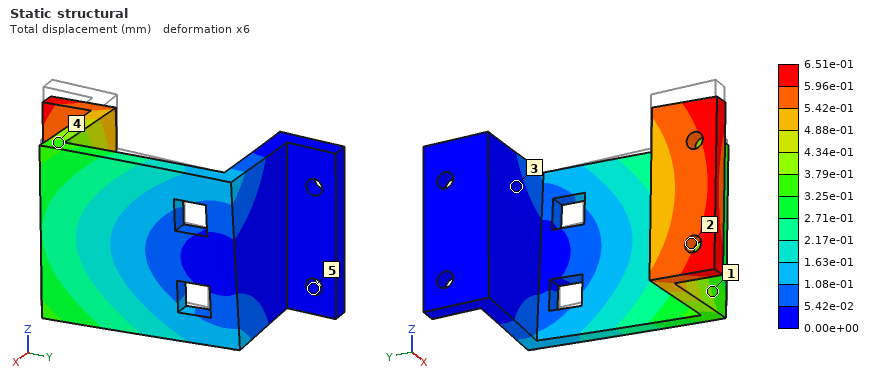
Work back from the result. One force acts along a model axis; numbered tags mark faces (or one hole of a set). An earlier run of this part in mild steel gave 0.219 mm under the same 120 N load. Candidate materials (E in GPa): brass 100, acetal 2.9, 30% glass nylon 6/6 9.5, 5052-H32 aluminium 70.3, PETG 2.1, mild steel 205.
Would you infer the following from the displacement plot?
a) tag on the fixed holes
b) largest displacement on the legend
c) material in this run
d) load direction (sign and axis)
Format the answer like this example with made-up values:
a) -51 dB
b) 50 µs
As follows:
a) 5
b) 6.51e-01 mm
c) 5052-H32 aluminium
d) -Z
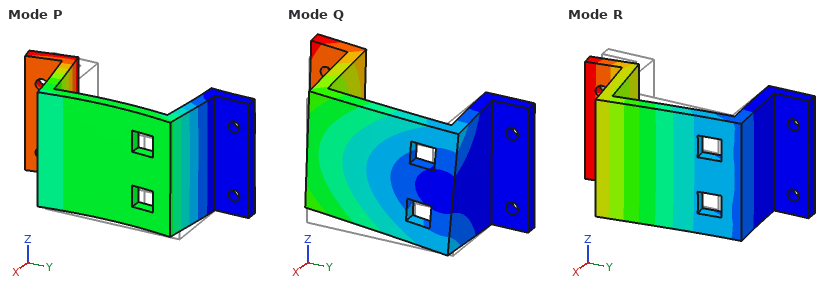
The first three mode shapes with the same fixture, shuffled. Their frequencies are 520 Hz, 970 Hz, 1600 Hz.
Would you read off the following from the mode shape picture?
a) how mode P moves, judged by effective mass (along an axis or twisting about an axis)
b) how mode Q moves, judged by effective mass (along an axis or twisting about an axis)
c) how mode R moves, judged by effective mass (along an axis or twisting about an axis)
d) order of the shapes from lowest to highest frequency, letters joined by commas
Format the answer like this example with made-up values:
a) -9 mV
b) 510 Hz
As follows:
a) along Y
b) along Z
c) along X
d) R, Q, P
